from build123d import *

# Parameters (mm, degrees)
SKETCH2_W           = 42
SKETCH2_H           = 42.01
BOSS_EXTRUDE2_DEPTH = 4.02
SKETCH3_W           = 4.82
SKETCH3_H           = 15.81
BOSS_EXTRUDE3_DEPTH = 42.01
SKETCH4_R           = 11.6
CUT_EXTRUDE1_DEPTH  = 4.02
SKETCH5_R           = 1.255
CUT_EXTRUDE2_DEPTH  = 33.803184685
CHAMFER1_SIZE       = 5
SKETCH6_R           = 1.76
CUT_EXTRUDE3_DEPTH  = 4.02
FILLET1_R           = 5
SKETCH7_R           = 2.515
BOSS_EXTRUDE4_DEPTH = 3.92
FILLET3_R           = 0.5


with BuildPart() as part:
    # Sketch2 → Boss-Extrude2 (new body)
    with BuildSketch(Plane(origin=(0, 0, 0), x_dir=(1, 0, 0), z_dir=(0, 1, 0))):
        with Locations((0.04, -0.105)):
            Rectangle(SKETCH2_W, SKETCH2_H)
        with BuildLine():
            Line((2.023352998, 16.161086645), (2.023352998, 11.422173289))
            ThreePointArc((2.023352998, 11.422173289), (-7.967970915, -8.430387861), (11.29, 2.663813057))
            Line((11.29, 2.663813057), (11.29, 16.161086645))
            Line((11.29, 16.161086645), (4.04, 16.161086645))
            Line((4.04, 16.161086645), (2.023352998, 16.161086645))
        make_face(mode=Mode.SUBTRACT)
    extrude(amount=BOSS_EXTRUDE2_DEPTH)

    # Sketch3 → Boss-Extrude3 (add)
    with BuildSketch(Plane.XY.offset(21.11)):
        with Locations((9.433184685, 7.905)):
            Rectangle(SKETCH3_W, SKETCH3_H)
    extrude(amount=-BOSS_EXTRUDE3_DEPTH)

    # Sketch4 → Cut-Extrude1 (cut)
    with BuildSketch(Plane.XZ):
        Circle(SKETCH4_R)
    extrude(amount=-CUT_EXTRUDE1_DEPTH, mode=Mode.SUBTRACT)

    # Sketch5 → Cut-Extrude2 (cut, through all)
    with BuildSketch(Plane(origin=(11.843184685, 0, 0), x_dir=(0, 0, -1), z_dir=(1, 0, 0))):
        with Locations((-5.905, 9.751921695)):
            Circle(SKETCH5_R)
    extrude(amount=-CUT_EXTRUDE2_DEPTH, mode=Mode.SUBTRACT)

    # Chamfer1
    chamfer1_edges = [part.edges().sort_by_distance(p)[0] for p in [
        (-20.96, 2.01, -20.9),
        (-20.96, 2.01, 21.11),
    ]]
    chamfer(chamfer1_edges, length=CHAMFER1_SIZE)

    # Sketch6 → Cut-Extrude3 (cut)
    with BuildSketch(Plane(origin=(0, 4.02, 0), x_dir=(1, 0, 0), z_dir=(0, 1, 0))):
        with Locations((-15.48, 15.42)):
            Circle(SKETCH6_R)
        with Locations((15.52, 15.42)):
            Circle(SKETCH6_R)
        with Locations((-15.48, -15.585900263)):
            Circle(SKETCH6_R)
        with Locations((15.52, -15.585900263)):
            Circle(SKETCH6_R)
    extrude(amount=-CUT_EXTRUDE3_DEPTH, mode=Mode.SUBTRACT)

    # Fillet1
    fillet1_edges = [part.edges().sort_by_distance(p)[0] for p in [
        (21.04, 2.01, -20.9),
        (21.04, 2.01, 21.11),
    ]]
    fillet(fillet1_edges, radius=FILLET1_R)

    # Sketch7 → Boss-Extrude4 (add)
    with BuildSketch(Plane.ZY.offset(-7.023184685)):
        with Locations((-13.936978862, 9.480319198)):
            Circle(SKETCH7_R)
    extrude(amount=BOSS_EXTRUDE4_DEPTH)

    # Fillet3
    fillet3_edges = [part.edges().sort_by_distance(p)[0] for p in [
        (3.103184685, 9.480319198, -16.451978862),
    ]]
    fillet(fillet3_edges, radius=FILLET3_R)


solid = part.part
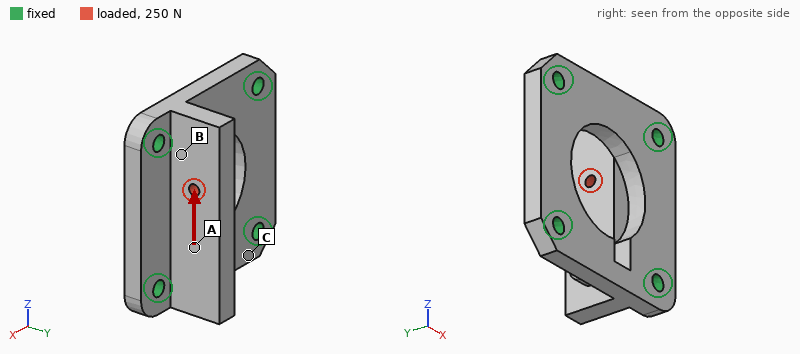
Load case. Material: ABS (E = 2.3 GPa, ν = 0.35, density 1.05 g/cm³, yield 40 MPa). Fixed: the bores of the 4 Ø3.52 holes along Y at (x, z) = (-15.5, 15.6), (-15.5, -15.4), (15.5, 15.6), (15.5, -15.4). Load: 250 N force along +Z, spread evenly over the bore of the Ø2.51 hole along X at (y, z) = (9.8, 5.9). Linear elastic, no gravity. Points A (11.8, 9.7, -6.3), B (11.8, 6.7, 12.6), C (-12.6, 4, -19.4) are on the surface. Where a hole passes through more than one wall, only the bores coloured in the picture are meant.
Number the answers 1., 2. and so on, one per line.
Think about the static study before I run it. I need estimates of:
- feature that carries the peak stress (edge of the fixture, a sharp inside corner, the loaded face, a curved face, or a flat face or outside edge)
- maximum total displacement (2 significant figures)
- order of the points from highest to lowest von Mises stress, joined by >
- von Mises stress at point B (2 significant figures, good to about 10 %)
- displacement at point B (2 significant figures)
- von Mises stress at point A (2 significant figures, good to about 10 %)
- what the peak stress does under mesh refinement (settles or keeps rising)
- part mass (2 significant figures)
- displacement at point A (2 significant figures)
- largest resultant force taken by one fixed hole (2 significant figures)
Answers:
1. edge of the fixture
2. 56 µm
3. B > A > C
4. 3.9 MPa
5. 27 µm
6. 2.4 MPa
7. keeps rising
8. 7.8 g
9. 30 µm
10. 140 N
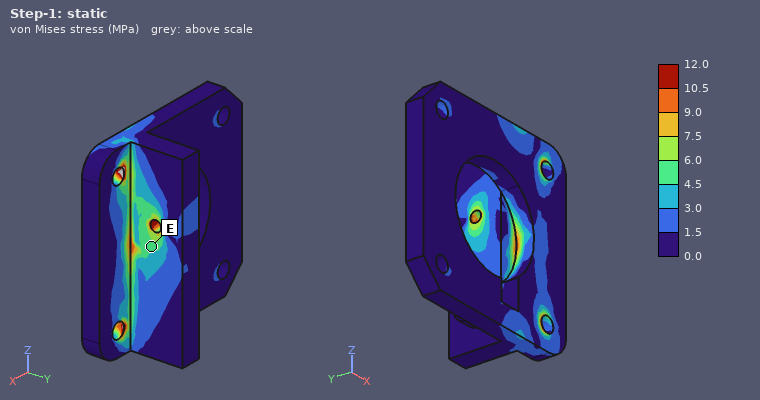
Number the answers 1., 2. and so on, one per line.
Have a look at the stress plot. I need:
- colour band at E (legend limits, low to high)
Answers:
1. 4.5 to 6.0 MPa
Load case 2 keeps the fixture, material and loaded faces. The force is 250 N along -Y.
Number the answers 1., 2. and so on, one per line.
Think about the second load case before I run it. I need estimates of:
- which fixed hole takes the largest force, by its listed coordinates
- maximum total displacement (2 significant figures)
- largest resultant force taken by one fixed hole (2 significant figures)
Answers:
1. (15.5, 15.6)
2. 0.17 mm
3. 160 N
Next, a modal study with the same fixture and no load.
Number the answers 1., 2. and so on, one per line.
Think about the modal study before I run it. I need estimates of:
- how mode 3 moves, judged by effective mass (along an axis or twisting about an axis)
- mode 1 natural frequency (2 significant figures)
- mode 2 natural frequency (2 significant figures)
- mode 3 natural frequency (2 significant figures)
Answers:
1. along Y
2. 2900 Hz
3. 4600 Hz
4. 6400 Hz
